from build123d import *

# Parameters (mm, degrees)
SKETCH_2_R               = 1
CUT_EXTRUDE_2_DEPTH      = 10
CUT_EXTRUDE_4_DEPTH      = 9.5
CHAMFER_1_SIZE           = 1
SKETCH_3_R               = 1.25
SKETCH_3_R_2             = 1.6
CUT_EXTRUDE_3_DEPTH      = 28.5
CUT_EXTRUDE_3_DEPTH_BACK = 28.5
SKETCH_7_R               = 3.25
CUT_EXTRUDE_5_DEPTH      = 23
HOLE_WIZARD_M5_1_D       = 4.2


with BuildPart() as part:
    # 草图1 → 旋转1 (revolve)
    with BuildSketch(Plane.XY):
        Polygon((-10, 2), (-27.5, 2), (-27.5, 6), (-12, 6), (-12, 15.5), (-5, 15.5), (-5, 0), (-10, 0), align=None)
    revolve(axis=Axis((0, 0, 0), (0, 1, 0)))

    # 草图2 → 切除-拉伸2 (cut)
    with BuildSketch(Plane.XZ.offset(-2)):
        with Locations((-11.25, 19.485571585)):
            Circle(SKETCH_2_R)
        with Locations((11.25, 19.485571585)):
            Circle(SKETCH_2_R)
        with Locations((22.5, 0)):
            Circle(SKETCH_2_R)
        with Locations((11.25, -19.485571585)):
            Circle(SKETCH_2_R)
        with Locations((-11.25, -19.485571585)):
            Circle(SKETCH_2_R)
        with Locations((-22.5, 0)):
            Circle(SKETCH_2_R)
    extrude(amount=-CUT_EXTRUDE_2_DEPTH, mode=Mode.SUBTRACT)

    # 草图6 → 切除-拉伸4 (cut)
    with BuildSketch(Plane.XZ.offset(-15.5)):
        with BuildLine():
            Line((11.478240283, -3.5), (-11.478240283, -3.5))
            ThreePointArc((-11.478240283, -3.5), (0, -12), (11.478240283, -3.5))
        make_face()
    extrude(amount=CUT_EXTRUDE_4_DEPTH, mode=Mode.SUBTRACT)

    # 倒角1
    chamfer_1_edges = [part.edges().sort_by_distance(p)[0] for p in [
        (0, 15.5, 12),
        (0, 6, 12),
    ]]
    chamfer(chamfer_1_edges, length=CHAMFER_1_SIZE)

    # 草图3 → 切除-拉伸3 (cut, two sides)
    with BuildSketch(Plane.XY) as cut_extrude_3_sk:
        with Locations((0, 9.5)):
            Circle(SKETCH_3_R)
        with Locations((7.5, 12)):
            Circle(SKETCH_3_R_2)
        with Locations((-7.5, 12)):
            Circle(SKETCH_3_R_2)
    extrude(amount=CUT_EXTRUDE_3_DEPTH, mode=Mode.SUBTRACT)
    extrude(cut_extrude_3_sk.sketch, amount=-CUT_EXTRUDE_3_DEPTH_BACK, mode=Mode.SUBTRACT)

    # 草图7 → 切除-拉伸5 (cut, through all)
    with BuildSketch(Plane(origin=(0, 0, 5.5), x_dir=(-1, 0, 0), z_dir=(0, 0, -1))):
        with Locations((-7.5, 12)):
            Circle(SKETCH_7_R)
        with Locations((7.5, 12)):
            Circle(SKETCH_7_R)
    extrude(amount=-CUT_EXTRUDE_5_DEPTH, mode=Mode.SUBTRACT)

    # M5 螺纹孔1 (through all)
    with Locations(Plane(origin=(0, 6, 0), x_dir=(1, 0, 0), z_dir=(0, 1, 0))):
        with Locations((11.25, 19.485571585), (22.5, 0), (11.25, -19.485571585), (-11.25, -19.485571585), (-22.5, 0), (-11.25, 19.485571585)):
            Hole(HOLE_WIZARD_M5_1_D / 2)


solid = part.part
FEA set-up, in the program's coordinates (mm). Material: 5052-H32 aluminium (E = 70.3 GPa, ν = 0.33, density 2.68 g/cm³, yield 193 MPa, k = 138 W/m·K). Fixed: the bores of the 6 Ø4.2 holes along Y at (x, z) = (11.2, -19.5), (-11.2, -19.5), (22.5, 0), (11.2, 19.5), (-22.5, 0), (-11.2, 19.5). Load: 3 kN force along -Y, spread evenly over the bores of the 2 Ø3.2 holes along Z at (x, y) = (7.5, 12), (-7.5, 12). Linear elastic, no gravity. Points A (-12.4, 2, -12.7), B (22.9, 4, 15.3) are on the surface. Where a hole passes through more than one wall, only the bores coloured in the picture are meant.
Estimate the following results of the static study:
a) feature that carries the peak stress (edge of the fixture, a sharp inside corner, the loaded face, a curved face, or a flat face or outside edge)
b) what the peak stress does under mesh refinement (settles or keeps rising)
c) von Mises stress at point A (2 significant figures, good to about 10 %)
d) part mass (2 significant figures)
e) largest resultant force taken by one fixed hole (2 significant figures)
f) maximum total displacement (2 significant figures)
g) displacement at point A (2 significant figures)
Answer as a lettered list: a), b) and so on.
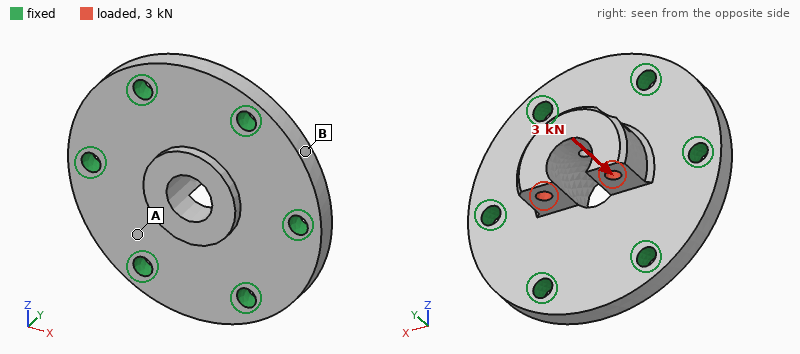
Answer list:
a) edge of the fixture
b) keeps rising
c) 24 MPa
d) 30 g
e) 680 N
f) 33 µm
g) 7.2 µm
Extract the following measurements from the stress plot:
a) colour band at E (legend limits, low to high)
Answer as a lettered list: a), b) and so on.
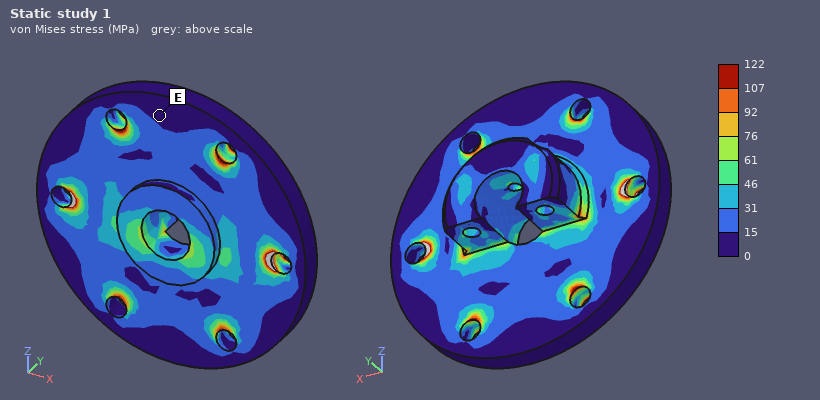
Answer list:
a) 0 to 15 MPa
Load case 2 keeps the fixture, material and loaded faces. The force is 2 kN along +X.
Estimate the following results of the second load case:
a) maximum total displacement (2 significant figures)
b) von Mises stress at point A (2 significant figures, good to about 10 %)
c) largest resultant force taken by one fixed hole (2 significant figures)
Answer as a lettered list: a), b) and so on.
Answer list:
a) 21 µm
b) 4.9 MPa
c) 650 N
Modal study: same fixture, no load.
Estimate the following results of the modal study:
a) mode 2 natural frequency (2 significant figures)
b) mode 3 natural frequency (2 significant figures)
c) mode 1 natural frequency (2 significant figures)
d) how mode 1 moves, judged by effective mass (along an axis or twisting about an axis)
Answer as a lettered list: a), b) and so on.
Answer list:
a) 25 kHz
b) 26 kHz
c) 17 kHz
d) along Y
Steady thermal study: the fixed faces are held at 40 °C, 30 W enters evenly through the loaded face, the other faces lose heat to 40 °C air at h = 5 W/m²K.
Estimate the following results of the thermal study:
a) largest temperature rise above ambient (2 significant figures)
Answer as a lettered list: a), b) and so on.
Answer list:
a) 21 K
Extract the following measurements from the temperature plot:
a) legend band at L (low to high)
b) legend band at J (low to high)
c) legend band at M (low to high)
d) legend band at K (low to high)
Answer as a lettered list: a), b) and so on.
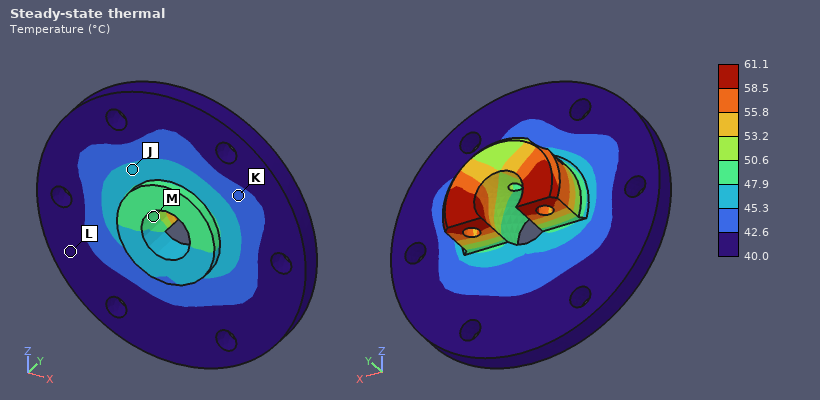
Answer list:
a) 40.0 to 42.6 °C
b) 45.3 to 47.9 °C
c) 47.9 to 50.6 °C
d) 42.6 to 45.3 °C
